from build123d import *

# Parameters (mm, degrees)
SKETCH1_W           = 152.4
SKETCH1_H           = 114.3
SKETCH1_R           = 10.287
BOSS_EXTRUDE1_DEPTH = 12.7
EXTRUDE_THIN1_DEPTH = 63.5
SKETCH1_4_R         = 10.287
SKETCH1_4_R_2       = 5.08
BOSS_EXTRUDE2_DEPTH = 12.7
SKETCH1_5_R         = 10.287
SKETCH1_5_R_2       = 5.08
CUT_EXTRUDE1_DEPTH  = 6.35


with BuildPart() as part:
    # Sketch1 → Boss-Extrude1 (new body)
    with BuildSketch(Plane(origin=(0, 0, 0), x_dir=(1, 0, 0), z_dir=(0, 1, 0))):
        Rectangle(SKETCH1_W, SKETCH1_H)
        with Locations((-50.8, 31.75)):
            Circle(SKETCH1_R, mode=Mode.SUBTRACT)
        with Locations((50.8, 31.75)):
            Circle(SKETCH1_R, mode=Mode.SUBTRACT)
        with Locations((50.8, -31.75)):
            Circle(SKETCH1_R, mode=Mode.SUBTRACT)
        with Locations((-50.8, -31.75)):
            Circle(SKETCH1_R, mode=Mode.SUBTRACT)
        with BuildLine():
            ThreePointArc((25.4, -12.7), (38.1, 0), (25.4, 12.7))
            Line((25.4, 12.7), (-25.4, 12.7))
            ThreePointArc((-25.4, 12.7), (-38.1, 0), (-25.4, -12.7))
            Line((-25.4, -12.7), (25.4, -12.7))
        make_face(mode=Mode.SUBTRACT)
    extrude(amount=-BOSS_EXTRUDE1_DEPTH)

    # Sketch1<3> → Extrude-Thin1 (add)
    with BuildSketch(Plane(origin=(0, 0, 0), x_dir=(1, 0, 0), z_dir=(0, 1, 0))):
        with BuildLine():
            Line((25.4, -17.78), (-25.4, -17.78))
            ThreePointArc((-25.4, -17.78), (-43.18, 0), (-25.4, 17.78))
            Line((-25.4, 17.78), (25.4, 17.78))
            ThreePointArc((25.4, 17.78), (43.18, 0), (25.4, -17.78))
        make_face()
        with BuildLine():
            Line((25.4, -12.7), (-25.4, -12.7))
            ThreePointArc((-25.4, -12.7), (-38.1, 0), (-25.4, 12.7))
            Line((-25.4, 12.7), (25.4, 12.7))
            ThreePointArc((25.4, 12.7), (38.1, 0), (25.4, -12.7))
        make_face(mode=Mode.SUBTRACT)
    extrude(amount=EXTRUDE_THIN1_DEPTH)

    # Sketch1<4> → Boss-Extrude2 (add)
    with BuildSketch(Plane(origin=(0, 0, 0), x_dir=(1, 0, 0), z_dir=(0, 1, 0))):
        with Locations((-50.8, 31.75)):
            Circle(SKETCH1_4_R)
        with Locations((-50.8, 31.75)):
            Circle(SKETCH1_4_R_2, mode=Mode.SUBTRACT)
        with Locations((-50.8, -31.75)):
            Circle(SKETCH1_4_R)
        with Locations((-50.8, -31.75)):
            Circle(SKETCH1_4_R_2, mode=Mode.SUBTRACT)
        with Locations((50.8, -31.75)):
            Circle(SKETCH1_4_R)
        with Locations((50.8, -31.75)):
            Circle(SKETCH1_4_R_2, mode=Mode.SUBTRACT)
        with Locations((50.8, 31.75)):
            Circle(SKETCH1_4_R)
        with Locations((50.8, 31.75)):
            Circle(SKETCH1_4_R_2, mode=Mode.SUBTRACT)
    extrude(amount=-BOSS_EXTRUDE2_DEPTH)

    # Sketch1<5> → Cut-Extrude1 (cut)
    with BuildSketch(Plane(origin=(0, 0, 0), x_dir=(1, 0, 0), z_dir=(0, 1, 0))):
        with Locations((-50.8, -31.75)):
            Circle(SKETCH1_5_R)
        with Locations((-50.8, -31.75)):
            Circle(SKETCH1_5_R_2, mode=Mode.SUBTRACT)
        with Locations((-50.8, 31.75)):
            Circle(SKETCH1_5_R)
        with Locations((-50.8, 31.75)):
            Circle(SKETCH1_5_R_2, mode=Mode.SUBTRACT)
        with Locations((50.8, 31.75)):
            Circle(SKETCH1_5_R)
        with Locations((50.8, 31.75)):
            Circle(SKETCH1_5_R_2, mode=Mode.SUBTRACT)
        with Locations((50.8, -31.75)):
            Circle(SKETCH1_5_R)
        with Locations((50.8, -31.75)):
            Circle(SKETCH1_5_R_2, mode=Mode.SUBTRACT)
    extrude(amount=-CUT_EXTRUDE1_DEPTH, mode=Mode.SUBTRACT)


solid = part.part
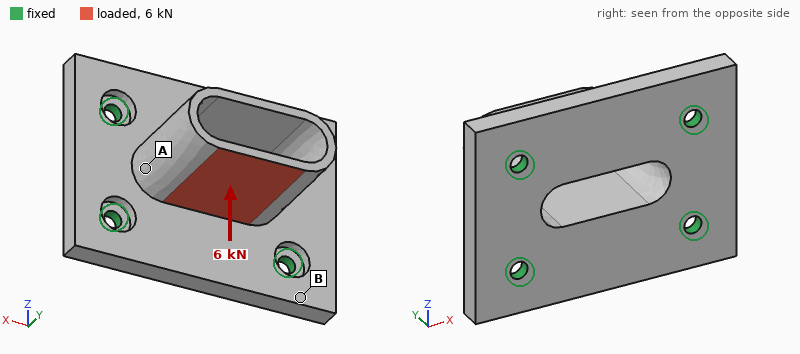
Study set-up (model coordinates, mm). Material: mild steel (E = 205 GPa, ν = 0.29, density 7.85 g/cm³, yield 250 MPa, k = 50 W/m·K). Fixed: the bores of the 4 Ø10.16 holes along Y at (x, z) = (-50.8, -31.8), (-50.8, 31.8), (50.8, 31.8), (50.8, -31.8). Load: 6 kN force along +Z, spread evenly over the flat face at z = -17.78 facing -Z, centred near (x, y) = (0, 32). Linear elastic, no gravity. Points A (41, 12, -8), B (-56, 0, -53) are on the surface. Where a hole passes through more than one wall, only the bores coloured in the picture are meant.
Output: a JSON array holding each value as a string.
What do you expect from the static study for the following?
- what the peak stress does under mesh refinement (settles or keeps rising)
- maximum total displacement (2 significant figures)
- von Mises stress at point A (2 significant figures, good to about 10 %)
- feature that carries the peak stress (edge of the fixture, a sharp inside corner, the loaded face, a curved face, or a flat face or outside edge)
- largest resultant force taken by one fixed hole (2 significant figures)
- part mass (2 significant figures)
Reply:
["keeps rising", "0.14 mm", "22 MPa", "edge of the fixture", "3.0 kN", "2.0 kg"]
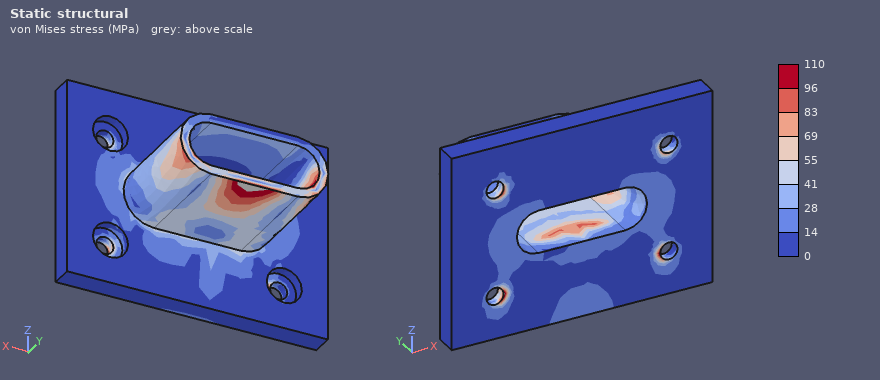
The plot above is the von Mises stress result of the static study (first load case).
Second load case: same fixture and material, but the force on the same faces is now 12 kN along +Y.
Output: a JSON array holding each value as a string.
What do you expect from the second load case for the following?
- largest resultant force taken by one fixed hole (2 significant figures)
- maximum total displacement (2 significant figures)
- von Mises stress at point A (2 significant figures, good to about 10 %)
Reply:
["6.7 kN", "81 µm", "25 MPa"]
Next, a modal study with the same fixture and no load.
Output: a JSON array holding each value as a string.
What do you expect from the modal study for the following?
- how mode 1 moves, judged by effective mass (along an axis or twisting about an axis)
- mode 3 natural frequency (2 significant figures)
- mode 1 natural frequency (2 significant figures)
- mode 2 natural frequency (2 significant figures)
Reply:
["along Z", "4200 Hz", "2700 Hz", "3800 Hz"]
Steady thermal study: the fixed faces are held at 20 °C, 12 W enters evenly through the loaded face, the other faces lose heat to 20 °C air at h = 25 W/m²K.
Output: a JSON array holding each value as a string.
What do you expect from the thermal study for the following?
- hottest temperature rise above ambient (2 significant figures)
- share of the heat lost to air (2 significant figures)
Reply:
["15 K", "39 %"]
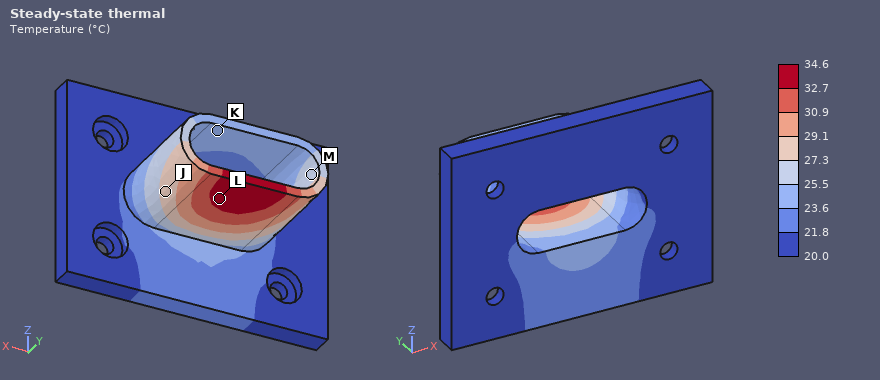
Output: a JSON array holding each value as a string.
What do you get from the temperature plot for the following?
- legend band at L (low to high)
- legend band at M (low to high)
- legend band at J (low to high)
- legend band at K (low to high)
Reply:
["32.7 to 34.6 °C", "25.5 to 27.3 °C", "27.3 to 29.1 °C", "23.6 to 25.5 °C"]
